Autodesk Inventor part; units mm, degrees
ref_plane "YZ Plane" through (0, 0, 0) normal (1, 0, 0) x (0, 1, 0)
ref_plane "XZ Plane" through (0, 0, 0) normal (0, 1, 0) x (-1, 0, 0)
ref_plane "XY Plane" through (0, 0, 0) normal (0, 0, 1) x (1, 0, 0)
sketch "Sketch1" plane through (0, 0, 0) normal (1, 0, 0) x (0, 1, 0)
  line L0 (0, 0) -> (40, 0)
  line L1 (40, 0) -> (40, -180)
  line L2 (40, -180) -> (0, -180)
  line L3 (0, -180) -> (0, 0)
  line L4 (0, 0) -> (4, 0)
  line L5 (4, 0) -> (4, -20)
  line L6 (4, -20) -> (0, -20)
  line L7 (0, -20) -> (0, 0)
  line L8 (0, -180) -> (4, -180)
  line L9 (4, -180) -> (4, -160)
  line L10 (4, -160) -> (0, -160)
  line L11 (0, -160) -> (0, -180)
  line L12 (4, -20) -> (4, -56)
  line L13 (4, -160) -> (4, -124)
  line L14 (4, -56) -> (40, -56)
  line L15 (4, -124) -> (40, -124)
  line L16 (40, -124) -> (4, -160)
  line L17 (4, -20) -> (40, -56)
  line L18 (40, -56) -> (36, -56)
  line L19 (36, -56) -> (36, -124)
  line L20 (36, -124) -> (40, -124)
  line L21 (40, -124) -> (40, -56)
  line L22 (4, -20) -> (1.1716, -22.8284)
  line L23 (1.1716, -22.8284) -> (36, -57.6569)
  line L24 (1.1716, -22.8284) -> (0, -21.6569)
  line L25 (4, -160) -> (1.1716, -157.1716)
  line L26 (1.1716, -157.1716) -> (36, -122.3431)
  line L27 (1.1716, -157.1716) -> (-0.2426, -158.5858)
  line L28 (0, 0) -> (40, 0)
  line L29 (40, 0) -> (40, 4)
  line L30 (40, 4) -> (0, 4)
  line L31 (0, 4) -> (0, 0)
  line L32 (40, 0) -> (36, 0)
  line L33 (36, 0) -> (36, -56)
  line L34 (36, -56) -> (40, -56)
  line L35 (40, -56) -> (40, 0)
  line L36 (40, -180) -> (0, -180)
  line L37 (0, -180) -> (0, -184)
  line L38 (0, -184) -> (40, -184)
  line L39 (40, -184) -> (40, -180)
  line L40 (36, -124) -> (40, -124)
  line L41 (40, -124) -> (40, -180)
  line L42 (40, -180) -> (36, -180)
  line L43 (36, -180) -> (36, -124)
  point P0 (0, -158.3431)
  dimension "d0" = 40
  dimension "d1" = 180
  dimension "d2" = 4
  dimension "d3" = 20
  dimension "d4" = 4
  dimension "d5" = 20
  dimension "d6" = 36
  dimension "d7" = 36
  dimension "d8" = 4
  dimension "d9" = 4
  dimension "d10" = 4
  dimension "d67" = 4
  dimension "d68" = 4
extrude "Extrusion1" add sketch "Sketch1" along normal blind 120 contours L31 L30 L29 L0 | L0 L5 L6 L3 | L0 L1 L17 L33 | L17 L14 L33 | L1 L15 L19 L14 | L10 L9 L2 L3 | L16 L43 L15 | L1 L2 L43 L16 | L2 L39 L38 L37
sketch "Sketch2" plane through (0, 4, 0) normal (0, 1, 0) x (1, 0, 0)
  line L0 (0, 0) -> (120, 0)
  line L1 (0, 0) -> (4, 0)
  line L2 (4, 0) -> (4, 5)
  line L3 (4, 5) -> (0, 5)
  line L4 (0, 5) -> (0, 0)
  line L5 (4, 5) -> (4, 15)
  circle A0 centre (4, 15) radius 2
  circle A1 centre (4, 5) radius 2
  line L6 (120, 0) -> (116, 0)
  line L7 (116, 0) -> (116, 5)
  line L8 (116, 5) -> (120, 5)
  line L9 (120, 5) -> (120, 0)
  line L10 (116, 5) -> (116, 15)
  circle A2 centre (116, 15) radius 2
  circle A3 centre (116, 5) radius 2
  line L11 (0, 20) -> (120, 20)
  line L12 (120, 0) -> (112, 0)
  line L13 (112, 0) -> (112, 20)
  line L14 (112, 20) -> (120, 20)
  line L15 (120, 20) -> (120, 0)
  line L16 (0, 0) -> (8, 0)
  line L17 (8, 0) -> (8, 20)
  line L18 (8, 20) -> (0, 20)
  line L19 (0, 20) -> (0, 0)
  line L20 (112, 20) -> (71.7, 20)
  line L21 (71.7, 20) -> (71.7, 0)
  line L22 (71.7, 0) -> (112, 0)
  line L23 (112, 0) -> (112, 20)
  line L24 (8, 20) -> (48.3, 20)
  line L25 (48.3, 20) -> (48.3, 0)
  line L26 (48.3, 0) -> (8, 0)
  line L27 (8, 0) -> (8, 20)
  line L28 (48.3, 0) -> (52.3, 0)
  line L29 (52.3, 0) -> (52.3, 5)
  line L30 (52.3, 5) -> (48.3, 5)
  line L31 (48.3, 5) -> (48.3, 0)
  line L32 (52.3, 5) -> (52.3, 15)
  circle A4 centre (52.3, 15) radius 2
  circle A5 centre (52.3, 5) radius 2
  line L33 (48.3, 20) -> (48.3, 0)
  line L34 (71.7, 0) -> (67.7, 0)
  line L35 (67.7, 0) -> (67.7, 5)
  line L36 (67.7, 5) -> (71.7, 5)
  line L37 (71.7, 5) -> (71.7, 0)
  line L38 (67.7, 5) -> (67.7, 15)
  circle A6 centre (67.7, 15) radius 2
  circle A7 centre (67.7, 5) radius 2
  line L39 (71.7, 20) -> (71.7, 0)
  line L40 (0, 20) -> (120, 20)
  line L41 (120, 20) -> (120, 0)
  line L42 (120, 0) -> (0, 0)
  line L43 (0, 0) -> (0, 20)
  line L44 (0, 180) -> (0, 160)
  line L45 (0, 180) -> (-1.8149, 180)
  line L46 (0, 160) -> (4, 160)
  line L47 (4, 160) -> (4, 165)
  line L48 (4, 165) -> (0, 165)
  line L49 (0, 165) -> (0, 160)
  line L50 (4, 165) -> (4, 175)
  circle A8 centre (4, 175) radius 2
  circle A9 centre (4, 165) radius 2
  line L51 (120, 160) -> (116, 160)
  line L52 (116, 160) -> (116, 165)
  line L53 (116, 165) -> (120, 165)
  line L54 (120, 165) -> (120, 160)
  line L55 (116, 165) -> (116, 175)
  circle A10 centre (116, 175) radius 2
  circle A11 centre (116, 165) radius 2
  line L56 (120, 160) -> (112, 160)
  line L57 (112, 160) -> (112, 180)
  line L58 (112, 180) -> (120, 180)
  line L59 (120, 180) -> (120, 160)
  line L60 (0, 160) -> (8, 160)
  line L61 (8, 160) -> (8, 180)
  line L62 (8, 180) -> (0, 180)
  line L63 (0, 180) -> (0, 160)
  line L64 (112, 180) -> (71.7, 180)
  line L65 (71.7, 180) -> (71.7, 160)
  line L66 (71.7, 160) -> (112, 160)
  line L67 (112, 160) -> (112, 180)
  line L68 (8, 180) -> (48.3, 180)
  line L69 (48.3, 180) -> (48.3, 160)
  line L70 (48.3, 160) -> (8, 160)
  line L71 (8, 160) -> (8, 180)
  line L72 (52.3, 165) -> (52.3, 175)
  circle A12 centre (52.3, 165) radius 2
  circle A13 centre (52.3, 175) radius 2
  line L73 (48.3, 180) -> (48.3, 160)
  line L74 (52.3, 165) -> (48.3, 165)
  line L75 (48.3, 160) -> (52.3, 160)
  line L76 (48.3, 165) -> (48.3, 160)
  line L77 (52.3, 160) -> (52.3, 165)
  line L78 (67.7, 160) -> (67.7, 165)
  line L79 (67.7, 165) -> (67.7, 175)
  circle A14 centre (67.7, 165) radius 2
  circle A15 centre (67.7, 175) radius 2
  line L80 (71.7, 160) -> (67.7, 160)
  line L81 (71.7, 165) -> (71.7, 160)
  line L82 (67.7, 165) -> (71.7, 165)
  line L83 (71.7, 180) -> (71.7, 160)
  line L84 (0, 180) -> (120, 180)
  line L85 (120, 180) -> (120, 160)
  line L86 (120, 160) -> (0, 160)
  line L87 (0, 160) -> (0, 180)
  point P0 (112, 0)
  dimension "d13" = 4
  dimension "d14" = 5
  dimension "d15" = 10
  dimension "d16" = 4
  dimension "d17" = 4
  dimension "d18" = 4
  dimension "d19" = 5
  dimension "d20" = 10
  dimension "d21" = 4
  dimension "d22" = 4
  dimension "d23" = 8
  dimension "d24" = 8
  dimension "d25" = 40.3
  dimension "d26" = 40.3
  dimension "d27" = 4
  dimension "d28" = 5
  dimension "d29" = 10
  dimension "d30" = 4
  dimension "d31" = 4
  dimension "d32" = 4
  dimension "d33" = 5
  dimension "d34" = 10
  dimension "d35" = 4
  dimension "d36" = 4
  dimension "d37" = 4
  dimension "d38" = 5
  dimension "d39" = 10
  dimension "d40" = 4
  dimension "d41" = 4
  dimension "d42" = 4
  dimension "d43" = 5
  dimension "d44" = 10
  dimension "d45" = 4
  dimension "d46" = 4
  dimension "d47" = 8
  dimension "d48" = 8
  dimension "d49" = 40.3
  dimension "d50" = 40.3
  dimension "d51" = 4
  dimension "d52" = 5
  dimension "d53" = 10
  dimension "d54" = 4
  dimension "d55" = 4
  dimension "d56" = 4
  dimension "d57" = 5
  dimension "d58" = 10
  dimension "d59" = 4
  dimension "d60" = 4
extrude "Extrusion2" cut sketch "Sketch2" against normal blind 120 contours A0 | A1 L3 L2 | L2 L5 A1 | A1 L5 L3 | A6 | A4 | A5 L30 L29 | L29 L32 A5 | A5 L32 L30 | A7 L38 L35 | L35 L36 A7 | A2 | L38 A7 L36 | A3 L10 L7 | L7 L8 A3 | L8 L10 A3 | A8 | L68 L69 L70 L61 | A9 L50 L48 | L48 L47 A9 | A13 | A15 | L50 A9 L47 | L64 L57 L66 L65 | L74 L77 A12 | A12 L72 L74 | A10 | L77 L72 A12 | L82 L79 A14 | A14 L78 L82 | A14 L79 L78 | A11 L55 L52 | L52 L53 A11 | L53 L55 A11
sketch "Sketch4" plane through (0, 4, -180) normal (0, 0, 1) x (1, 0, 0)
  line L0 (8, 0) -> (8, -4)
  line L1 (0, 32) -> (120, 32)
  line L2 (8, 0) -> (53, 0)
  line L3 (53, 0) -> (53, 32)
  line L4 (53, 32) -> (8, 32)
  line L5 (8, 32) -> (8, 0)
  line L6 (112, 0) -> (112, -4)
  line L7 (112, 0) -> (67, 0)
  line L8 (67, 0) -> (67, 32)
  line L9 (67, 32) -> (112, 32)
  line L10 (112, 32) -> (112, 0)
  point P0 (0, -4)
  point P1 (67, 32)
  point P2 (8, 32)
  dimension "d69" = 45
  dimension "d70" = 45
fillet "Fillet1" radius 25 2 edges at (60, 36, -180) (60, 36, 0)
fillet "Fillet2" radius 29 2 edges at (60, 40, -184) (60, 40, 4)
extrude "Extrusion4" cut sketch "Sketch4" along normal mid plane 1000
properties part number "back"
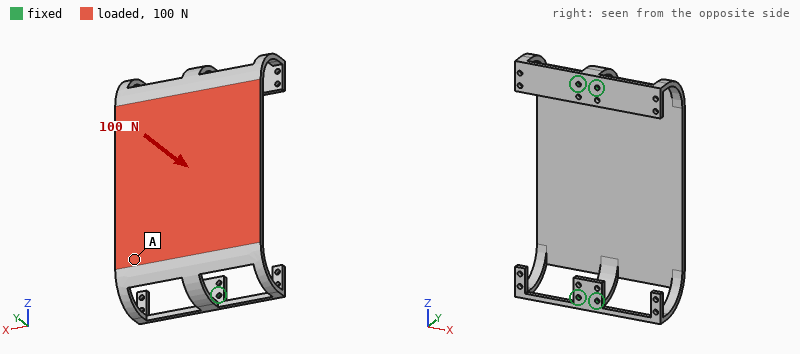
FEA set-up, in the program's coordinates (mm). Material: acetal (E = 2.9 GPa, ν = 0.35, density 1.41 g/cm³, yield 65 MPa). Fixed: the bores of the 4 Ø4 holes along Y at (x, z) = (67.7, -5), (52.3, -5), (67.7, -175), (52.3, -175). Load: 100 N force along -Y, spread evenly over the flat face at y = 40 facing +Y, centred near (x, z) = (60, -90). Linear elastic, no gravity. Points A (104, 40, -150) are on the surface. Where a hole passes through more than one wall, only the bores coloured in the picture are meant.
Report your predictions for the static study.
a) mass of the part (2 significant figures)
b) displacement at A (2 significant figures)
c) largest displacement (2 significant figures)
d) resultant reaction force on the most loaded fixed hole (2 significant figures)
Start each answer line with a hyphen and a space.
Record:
- 140 g
- 1.1 mm
- 2.5 mm
- 39 N
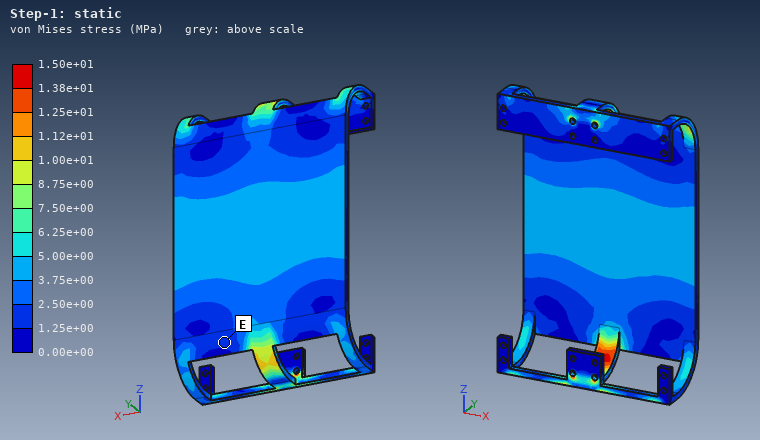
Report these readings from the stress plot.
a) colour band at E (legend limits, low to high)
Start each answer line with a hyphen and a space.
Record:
- 1.25e+00 to 2.50e+00 MPa
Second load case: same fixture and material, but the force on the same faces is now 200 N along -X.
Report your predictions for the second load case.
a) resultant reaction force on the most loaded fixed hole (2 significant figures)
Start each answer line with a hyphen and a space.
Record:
- 230 N
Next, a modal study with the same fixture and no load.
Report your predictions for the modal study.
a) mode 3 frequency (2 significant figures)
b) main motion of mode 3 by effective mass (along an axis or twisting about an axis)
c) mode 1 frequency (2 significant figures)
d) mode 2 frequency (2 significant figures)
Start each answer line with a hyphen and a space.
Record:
- 140 Hz
- along Z
- 120 Hz
- 120 Hz
